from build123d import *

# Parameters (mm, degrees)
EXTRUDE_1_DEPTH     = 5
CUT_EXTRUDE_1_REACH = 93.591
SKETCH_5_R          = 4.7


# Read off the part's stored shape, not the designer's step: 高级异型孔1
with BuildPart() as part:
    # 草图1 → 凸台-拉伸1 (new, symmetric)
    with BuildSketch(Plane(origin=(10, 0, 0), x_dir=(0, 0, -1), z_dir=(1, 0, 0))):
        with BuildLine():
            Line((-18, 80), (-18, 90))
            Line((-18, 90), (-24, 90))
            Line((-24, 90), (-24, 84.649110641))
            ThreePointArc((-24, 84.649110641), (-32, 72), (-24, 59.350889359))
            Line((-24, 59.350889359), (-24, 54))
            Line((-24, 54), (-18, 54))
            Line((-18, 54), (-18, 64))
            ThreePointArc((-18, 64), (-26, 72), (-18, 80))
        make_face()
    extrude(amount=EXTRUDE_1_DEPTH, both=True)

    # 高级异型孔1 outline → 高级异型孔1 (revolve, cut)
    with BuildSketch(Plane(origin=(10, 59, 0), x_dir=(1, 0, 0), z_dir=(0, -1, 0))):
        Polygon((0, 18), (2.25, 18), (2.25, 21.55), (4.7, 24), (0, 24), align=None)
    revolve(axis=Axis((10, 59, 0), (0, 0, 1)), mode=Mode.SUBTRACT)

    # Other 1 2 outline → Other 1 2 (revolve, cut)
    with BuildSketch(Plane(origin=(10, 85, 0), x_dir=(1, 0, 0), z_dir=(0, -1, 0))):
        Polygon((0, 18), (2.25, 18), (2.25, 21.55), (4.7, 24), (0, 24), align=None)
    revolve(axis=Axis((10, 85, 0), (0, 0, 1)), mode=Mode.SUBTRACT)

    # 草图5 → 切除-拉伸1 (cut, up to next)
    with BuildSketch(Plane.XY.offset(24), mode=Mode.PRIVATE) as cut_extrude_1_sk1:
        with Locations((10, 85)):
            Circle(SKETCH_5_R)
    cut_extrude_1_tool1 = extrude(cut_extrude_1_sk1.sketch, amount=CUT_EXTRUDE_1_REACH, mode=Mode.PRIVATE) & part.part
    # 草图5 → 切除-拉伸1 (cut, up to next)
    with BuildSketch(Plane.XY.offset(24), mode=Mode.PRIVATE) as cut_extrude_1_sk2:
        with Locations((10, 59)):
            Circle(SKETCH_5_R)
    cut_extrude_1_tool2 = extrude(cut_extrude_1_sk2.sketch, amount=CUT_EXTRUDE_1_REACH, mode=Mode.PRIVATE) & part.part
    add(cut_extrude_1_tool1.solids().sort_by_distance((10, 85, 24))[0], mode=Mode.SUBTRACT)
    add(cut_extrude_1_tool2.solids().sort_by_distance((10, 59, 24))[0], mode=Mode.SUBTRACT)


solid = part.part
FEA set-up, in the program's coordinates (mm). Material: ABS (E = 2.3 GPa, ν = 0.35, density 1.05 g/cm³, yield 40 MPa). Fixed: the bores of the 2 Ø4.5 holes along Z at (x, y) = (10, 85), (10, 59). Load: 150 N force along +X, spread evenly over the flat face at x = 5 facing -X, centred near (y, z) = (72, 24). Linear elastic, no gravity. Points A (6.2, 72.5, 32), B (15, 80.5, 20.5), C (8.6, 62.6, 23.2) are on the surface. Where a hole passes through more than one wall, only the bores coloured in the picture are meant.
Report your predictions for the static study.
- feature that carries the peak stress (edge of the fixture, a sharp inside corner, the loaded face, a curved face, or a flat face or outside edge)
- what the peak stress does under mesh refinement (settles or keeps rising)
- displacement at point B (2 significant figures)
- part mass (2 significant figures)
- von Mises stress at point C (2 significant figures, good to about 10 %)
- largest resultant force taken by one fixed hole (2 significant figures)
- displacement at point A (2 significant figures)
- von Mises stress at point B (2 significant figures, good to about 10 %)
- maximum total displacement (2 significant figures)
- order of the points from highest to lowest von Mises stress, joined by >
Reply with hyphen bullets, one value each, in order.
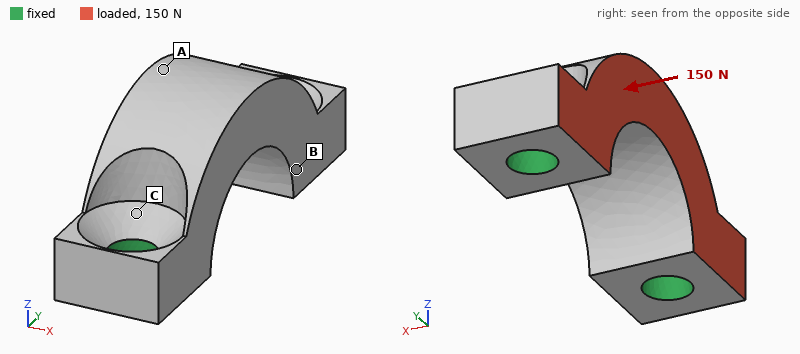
- edge of the fixture
- keeps rising
- 21 µm
- 2.2 g
- 5.4 MPa
- 75 N
- 79 µm
- 3.1 MPa
- 81 µm
- C > B > A
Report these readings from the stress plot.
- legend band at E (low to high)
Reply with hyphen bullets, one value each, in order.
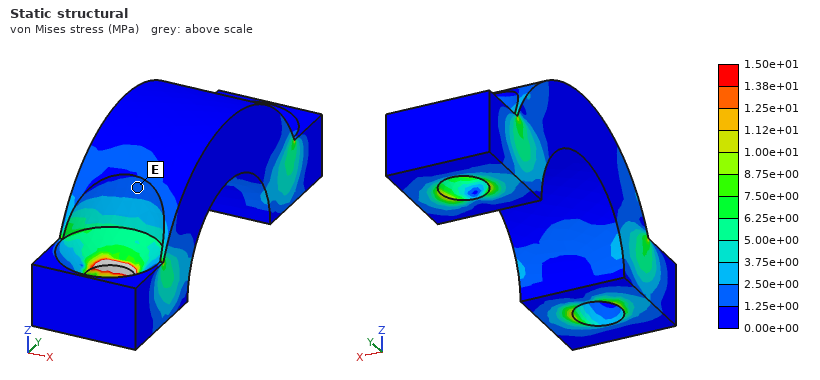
- 1.25e+00 to 2.50e+00 MPa
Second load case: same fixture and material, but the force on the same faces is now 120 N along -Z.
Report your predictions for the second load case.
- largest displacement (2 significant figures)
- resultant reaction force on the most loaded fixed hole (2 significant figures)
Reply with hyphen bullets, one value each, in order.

- 56 µm
- 63 N
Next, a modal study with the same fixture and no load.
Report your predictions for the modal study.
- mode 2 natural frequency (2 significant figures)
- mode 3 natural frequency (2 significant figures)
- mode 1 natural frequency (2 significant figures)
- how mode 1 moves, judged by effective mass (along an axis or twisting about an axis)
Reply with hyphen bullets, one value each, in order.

- 12 kHz
- 12 kHz
- 5200 Hz
- along X
